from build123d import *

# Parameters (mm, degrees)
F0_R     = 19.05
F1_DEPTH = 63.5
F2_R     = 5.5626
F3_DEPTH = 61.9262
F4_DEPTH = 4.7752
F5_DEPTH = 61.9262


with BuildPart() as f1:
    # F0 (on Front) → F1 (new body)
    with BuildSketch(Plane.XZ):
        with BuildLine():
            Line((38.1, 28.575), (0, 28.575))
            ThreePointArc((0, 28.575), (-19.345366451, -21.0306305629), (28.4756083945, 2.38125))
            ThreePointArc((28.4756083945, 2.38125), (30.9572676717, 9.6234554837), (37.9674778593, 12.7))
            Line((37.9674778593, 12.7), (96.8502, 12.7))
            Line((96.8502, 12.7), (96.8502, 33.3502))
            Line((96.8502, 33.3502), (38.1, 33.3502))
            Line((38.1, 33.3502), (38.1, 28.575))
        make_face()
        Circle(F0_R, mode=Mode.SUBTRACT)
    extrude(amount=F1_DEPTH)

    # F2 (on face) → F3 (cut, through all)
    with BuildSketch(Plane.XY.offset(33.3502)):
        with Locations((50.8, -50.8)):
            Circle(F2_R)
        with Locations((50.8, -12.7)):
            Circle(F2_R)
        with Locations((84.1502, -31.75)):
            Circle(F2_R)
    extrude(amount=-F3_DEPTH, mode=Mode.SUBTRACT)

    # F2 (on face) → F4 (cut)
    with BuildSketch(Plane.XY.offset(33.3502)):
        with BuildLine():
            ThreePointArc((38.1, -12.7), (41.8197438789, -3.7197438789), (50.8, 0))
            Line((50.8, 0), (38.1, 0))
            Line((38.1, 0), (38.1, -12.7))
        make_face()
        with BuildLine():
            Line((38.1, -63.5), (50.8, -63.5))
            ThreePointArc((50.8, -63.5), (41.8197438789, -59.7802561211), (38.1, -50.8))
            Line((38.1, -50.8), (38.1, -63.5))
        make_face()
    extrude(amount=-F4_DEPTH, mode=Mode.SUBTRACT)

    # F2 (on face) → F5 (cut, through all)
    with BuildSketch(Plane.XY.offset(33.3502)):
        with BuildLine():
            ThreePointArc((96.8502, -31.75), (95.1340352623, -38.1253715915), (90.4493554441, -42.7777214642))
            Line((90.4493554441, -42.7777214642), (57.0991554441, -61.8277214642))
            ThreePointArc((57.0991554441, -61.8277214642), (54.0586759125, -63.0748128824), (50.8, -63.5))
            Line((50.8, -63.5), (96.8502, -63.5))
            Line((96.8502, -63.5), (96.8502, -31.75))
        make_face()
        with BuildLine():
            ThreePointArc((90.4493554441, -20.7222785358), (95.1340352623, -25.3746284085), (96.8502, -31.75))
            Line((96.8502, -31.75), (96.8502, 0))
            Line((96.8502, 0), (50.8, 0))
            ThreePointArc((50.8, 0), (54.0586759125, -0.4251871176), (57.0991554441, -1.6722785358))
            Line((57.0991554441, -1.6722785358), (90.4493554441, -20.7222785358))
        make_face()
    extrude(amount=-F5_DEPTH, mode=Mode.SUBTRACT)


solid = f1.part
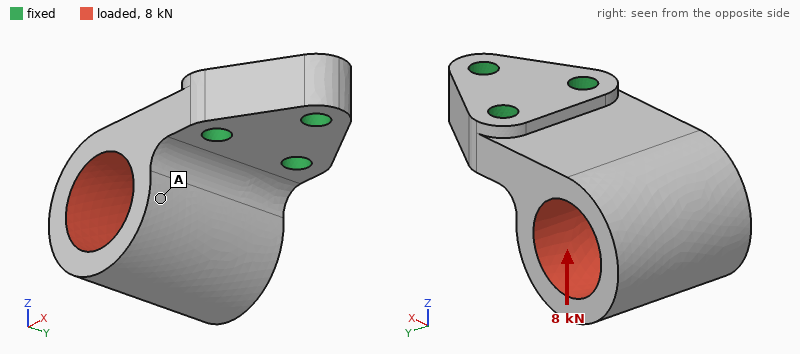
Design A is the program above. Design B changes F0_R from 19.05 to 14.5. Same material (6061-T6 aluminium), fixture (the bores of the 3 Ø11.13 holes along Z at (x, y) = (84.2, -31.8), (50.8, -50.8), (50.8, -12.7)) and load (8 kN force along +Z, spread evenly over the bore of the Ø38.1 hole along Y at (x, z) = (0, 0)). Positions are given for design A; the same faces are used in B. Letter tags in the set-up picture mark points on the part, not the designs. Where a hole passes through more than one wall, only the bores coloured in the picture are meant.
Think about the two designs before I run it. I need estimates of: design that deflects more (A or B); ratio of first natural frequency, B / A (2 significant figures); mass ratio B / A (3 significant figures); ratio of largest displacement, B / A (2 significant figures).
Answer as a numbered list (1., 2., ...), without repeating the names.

1. A
2. 0.96
3. 1.19
4. 0.85
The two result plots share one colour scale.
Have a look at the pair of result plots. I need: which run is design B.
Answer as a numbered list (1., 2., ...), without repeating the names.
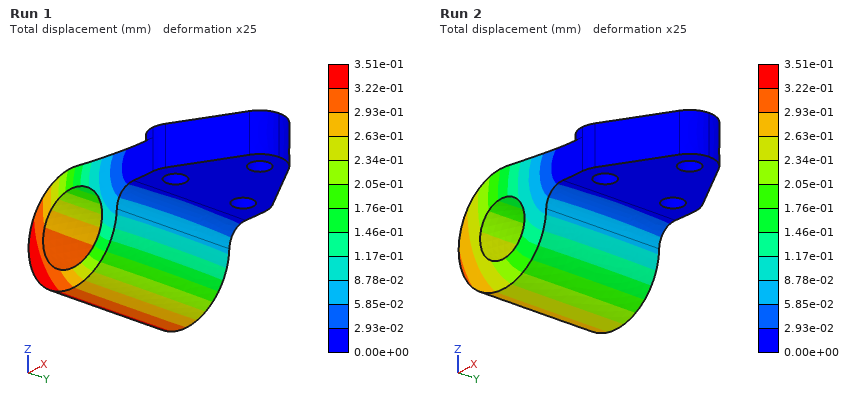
1. Run 2
